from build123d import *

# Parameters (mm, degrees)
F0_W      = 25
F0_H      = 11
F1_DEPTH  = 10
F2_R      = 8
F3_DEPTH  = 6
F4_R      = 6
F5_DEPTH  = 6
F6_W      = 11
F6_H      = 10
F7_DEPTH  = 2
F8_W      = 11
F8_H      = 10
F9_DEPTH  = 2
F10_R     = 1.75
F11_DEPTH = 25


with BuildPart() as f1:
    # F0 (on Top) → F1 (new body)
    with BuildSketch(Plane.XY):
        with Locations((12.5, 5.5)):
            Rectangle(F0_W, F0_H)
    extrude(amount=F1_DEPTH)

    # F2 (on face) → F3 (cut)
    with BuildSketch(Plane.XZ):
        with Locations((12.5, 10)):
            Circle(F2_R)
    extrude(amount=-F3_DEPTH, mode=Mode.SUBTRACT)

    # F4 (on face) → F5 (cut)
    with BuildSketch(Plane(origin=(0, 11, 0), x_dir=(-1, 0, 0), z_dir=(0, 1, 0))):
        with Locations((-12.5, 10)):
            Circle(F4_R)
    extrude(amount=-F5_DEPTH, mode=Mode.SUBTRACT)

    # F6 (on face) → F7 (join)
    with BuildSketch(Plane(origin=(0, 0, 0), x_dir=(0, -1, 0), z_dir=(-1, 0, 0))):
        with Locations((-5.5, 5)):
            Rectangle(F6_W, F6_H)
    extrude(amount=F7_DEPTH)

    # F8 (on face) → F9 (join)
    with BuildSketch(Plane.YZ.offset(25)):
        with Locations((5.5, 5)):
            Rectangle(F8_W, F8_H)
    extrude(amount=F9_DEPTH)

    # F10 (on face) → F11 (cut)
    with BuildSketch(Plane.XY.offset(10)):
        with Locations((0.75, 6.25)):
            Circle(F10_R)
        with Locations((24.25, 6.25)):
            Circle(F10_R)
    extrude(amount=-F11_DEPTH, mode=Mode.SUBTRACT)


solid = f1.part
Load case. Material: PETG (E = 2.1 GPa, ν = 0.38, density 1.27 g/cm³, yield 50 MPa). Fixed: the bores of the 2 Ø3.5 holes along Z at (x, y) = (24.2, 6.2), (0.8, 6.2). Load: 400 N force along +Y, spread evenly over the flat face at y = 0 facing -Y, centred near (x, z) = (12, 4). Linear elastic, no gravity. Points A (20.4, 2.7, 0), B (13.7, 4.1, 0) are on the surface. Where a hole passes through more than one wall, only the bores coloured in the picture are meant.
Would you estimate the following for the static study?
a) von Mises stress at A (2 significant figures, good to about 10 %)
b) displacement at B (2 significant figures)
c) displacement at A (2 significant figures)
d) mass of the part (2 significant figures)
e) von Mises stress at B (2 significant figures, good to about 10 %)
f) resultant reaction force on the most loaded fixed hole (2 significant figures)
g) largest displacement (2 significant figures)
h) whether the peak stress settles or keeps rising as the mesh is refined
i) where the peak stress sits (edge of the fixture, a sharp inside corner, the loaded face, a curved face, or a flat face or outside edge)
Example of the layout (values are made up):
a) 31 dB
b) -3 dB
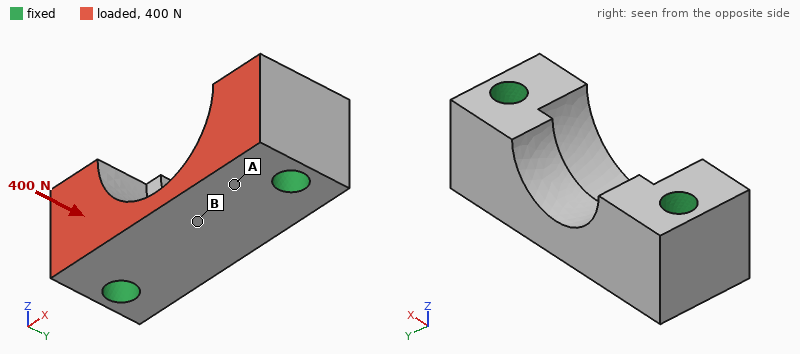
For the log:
a) 2.9 MPa
b) 26 µm
c) 13 µm
d) 2.7 g
e) 1.3 MPa
f) 200 N
g) 32 µm
h) keeps rising
i) edge of the fixture
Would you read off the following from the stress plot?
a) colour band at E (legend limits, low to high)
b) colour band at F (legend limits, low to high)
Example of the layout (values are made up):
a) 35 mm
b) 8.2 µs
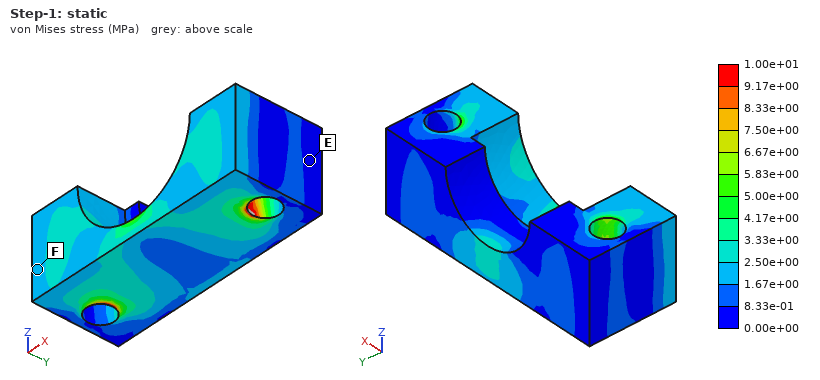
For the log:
a) 0.00e+00 to 8.33e-01 MPa
b) 1.67e+00 to 2.50e+00 MPa
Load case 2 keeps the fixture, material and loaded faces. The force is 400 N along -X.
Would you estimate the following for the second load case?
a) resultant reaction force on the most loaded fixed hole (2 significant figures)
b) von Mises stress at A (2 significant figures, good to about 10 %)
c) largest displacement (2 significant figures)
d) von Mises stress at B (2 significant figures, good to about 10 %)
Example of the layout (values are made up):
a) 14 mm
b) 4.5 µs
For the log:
a) 210 N
b) 4.9 MPa
c) 38 µm
d) 4.6 MPa
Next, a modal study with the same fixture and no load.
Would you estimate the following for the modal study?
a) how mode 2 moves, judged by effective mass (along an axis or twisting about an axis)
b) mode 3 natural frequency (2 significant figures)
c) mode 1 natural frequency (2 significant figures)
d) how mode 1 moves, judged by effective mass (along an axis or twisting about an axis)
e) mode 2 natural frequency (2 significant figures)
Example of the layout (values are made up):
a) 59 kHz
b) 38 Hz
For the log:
a) along Z
b) 21 kHz
c) 13 kHz
d) along Y
e) 16 kHz
